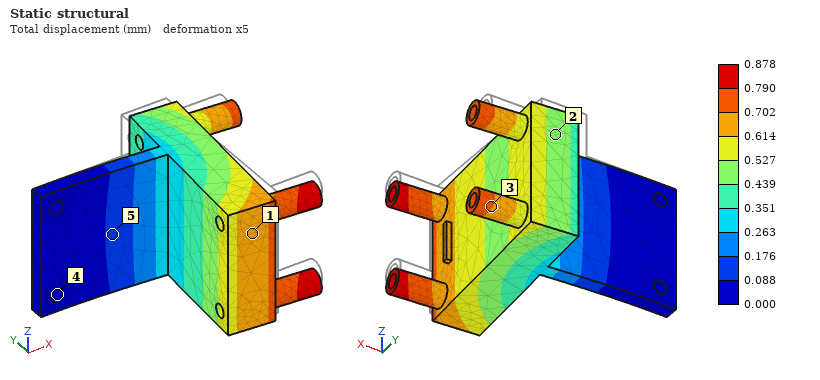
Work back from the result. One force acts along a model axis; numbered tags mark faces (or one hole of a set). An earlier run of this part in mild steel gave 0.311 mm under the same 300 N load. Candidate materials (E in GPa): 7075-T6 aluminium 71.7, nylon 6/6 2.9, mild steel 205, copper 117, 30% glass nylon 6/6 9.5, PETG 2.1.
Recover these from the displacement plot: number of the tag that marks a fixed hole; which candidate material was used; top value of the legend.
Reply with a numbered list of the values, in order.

1. 4
2. 7075-T6 aluminium
3. 0.878 mm
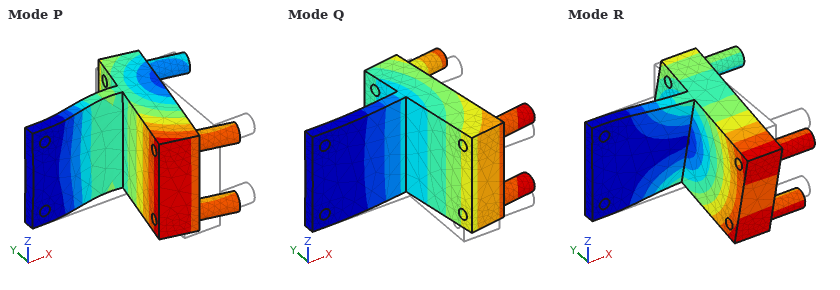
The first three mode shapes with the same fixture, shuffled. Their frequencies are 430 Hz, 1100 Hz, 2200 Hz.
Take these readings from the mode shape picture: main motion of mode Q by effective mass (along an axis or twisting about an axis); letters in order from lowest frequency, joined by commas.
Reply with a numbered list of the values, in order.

1. along Y
2. Q, R, P
